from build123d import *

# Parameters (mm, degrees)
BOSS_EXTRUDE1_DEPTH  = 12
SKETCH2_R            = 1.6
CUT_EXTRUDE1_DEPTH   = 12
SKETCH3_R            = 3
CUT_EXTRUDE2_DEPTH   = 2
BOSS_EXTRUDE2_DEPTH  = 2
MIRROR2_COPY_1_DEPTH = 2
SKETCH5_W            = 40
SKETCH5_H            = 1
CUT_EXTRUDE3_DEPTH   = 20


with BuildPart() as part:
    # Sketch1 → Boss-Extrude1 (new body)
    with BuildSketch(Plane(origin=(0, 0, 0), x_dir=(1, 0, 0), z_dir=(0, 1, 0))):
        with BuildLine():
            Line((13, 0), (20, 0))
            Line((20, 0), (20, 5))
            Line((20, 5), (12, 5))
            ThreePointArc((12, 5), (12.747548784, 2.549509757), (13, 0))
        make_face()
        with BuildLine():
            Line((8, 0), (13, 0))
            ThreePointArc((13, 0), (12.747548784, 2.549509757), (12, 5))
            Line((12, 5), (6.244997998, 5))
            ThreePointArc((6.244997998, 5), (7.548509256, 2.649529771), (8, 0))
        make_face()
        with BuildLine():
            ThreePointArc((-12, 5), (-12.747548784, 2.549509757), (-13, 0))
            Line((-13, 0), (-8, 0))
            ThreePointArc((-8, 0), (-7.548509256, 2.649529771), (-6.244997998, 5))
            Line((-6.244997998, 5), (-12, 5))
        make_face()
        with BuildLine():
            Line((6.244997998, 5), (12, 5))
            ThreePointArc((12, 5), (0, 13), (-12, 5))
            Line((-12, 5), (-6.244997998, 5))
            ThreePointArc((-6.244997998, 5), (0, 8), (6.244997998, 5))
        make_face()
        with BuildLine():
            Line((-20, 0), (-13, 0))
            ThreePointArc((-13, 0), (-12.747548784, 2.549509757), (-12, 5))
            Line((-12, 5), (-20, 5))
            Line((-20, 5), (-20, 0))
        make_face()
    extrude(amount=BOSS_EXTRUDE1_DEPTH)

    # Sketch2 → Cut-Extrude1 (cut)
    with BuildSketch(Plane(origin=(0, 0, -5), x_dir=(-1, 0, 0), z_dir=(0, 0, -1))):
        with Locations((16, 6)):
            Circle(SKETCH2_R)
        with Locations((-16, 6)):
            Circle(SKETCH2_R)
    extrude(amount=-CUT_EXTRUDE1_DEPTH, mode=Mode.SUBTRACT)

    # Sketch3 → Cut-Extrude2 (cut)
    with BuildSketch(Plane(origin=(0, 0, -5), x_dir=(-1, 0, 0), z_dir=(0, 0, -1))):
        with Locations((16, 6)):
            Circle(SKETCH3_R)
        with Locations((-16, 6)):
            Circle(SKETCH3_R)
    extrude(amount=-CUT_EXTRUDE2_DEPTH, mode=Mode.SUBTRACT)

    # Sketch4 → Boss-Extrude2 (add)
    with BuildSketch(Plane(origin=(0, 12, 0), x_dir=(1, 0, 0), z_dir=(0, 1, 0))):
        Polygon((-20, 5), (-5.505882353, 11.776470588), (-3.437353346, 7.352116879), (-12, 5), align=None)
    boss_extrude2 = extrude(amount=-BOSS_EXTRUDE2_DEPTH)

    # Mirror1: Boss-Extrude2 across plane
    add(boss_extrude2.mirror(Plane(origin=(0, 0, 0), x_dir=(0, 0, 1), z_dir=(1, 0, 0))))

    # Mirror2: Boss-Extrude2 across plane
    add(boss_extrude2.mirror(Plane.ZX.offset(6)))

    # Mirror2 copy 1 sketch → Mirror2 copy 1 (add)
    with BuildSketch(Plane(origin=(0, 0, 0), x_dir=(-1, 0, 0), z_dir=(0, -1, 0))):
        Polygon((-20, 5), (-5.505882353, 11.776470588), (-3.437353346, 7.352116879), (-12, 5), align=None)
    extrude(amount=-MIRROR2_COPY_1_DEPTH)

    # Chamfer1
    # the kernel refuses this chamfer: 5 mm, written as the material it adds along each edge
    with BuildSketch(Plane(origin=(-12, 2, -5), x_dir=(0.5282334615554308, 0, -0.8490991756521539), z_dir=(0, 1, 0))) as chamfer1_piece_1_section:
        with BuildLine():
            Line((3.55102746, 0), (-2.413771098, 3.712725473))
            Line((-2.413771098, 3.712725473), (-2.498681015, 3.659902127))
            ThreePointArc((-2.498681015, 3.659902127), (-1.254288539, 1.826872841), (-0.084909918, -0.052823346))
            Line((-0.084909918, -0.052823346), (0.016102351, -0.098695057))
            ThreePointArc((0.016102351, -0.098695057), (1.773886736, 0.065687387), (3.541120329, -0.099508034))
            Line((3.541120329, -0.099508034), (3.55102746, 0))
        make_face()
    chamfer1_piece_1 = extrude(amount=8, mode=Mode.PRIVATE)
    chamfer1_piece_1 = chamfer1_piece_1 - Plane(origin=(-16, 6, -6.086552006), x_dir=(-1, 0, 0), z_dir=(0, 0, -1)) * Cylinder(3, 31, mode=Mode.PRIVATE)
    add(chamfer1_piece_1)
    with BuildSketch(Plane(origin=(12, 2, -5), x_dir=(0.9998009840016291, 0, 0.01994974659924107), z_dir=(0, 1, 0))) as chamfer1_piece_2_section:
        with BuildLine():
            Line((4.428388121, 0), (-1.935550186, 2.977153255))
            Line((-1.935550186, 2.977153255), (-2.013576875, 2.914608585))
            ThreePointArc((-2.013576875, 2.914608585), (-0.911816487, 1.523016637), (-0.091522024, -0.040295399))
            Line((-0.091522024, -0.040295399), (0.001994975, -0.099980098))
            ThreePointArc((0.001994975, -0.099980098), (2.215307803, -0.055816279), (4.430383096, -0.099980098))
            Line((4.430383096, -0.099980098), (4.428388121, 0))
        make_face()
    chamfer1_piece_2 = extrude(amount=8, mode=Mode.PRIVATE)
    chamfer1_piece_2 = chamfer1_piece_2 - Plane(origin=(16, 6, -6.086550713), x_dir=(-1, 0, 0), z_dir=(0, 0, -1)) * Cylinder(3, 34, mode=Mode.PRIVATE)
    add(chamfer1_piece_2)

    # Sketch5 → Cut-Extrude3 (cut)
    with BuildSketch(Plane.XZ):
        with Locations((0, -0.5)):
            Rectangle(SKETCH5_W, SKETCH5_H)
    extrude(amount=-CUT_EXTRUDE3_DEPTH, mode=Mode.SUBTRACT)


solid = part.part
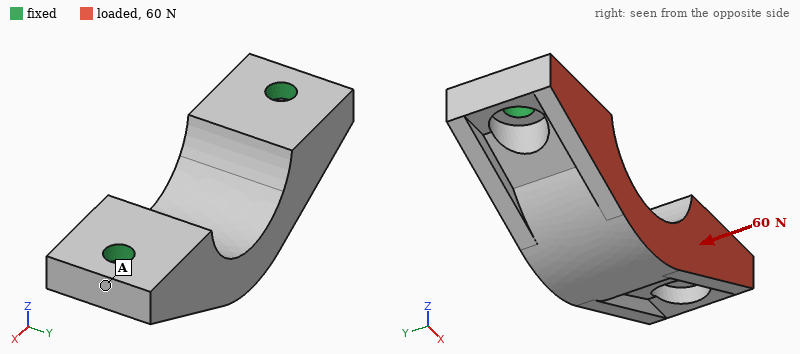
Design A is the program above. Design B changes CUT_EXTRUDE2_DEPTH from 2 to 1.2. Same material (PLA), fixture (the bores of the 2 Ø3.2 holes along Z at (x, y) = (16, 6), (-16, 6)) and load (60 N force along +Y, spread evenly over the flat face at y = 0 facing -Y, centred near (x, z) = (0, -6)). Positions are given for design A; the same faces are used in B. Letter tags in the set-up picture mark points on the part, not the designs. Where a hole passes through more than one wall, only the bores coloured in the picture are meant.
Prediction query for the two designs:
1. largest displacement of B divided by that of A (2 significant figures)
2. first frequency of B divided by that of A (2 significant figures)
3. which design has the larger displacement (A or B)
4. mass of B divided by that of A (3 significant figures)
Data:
0.62
1.3
A
1.01
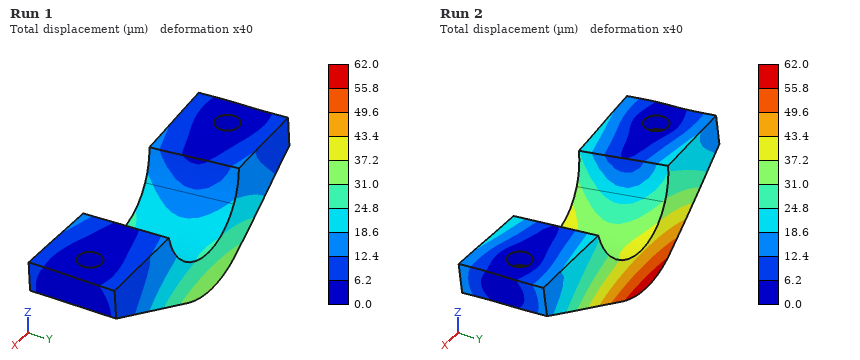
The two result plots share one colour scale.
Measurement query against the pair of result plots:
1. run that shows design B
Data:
Run 1
